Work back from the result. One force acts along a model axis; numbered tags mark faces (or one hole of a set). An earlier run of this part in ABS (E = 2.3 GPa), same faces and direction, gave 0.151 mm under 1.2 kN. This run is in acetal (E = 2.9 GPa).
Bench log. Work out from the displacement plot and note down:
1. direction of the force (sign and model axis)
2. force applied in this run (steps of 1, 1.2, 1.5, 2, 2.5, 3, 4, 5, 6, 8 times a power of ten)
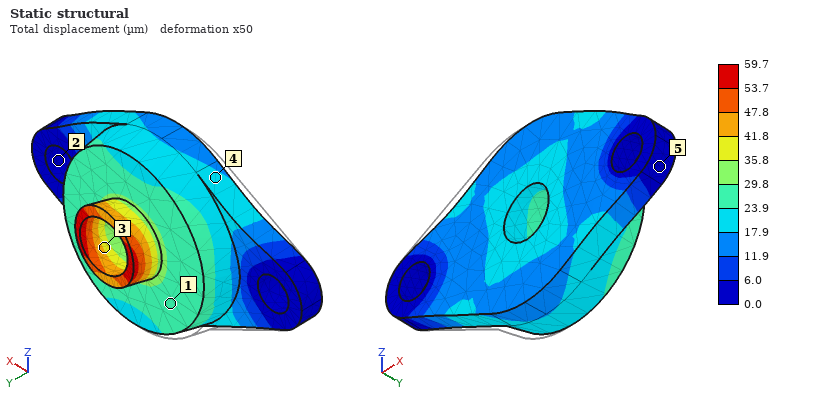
+X
600 N
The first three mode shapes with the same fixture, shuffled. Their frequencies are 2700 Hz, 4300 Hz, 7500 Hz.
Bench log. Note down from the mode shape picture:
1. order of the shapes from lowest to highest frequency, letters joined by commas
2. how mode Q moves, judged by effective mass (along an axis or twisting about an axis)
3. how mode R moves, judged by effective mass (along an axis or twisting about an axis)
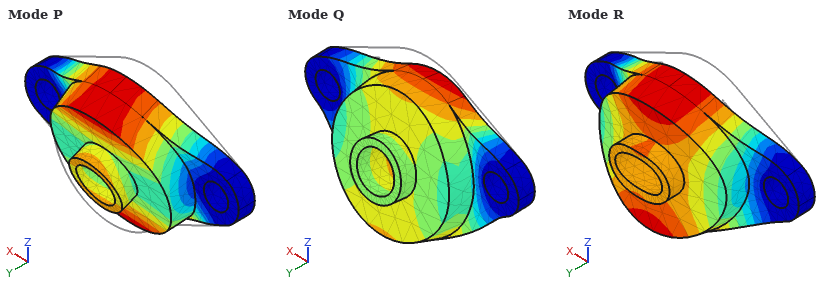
P, R, Q
along Z
along Y
